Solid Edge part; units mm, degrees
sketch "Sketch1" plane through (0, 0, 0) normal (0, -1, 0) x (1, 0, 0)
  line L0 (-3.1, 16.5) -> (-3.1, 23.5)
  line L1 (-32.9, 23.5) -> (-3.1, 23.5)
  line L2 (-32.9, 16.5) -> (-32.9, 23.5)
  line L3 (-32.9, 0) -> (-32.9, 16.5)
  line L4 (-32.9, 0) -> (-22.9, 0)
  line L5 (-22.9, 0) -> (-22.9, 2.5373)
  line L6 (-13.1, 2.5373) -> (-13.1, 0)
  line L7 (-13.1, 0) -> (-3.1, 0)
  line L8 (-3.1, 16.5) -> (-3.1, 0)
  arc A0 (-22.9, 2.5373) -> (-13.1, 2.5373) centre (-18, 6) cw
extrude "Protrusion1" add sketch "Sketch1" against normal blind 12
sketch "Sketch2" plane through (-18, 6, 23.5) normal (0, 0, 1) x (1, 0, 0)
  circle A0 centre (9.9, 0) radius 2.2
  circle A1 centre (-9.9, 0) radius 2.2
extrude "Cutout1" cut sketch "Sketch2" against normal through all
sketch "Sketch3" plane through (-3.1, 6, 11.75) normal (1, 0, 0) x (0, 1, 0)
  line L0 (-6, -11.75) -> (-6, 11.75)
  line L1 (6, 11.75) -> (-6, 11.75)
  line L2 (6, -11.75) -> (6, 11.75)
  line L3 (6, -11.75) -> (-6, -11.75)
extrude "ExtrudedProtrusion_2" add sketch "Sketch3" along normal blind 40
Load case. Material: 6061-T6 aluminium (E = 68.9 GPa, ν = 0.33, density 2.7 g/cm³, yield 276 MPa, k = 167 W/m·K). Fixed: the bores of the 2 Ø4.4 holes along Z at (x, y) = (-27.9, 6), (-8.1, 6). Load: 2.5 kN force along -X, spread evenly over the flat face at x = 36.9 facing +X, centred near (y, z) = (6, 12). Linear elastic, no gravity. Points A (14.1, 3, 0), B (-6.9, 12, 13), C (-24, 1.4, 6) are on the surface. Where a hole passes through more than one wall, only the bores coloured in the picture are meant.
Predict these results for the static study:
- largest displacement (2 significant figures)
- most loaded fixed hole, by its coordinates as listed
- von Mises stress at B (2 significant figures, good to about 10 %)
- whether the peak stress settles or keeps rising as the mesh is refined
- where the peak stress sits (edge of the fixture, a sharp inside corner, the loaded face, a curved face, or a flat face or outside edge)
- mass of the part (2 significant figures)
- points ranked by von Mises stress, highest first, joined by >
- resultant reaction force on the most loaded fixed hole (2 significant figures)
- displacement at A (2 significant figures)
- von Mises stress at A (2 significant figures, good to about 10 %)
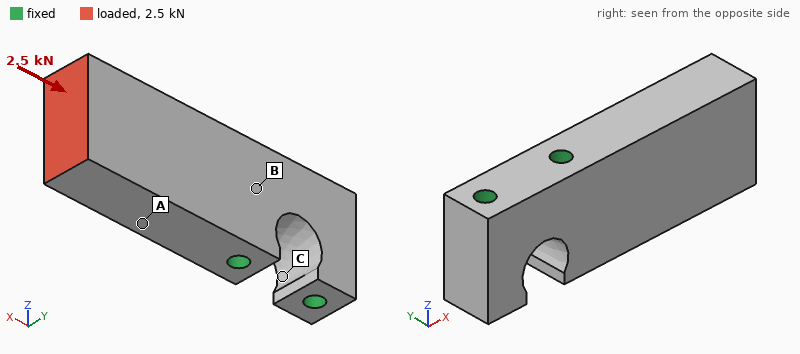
5.8 µm
(-8.1, 6)
4.3 MPa
keeps rising
edge of the fixture
47 g
A > B > C
2.4 kN
2.9 µm
8.7 MPa
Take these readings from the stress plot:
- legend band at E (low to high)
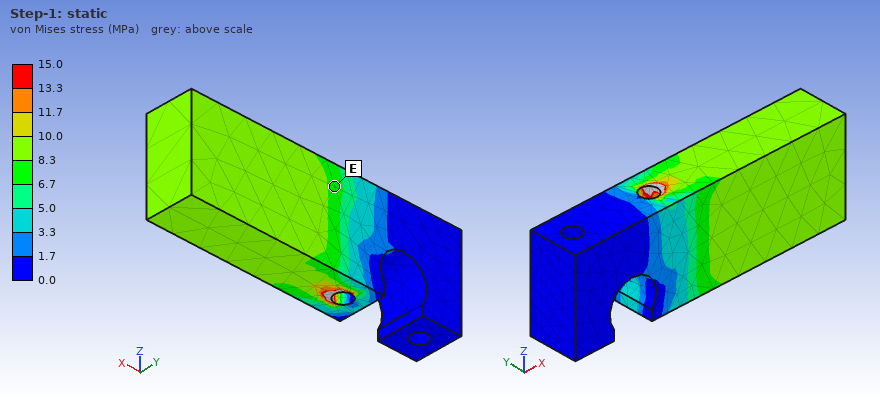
6.7 to 8.3 MPa
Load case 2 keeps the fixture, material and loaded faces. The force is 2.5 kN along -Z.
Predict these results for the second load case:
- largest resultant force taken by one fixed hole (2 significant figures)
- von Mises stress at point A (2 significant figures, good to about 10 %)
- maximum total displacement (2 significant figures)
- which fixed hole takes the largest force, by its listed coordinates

2.7 kN
52 MPa
0.11 mm
(-8.1, 6)
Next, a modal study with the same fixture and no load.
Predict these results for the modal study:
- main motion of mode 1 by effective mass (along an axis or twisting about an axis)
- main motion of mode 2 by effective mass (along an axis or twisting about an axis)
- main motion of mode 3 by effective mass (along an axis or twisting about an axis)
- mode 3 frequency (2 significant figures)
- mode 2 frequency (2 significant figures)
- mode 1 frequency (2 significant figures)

along Y
along Z
twisting about X
14 kHz
8000 Hz
4100 Hz
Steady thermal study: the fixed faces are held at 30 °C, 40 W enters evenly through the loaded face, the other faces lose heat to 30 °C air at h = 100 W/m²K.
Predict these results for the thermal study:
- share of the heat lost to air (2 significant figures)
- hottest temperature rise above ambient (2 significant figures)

13 %
34 K
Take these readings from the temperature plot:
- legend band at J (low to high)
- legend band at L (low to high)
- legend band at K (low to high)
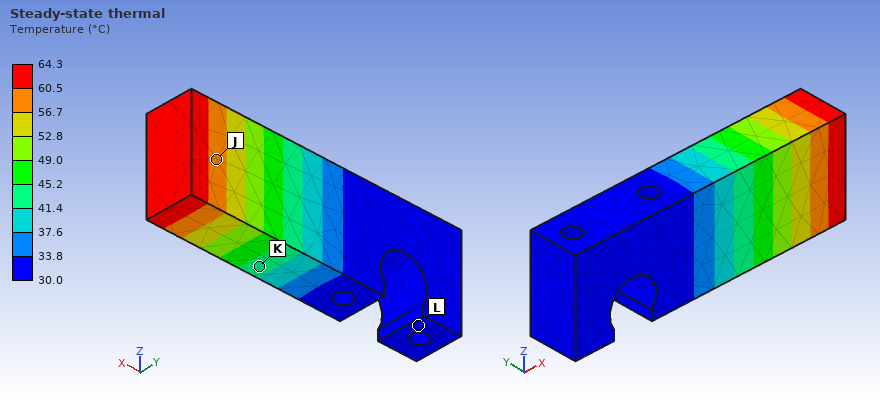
56.7 to 60.5 °C
30.0 to 33.8 °C
41.4 to 45.2 °C
